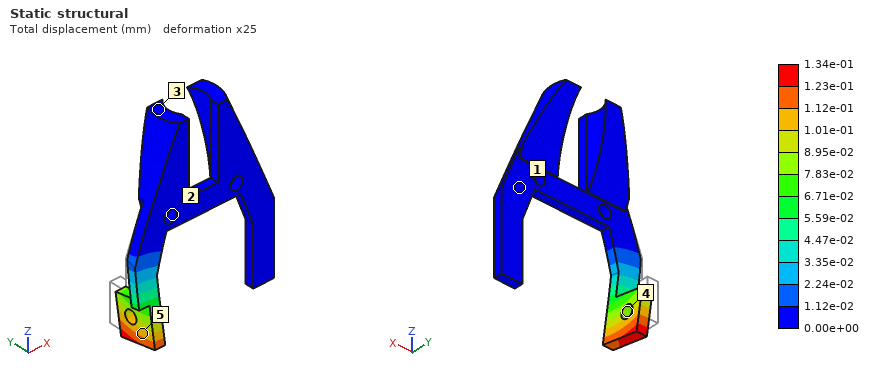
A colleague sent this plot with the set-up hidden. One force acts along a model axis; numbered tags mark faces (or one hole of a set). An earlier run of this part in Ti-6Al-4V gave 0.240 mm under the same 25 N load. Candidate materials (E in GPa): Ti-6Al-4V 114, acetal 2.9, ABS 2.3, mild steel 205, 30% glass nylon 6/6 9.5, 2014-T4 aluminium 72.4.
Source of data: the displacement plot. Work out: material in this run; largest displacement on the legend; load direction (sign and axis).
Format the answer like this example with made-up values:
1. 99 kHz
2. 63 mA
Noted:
1. mild steel
2. 1.34e-01 mm
3. -Y
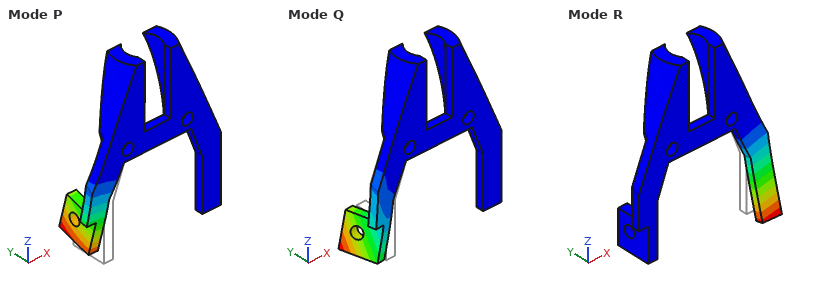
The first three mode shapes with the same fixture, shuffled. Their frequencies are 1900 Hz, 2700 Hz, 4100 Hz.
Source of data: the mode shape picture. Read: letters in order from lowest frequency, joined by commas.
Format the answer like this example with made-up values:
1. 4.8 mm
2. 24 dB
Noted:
1. P, R, Q
